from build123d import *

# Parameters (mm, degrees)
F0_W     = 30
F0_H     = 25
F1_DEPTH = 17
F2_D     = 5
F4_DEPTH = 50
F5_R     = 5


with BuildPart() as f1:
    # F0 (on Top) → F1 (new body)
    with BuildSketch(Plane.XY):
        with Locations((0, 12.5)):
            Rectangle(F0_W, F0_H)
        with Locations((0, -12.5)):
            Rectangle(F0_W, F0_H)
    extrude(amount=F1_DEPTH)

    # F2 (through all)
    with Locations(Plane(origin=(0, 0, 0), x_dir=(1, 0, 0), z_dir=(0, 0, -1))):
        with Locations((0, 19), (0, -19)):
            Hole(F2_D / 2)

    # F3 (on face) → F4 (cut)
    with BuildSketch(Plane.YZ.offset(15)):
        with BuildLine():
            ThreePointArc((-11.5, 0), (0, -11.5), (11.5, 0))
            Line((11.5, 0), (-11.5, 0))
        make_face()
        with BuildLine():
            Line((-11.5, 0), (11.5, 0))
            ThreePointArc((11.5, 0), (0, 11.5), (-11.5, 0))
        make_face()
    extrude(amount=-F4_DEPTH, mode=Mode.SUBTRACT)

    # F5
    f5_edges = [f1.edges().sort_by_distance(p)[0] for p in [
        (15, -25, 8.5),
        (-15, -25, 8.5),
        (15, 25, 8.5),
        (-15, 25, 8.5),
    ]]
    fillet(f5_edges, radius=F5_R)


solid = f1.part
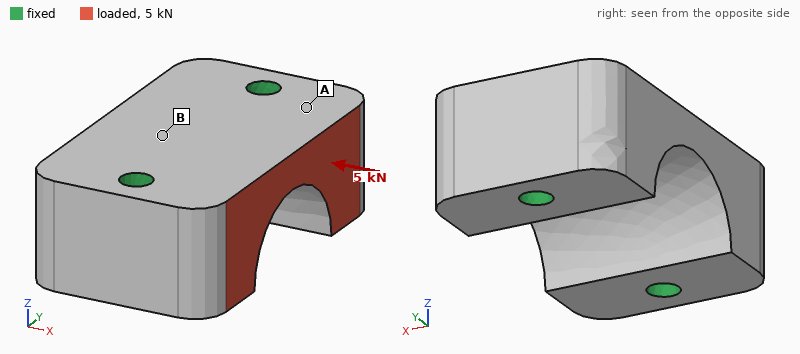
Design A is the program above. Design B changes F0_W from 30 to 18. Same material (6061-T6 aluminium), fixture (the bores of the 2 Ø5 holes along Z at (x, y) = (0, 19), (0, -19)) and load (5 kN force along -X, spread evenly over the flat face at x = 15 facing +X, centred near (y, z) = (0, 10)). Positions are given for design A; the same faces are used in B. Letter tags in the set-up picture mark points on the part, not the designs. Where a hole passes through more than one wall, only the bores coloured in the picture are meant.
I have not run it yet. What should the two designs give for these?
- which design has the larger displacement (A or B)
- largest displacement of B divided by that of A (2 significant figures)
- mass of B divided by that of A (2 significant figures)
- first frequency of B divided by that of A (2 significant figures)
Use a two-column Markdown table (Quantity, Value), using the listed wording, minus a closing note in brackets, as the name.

| Quantity | Value |
|---|---|
| which design has the larger displacement | B |
| largest displacement of B divided by that of A | 1.3 |
| mass of B divided by that of A | 0.58 |
| first frequency of B divided by that of A | 1.2 |
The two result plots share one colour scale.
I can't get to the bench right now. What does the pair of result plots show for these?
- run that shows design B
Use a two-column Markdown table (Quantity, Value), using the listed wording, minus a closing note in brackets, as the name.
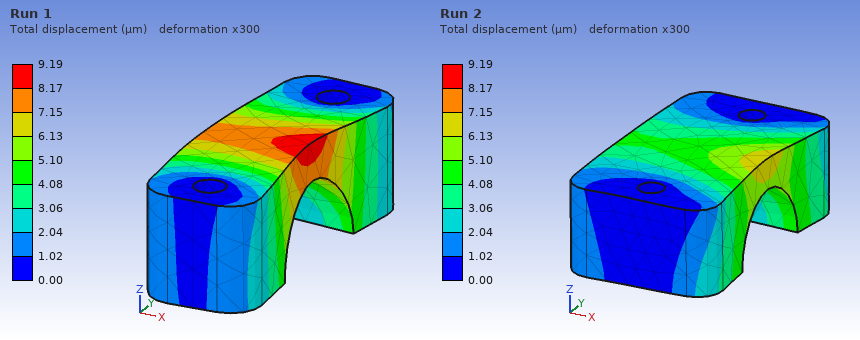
| Quantity | Value |
|---|---|
| run that shows design B | Run 1 |
